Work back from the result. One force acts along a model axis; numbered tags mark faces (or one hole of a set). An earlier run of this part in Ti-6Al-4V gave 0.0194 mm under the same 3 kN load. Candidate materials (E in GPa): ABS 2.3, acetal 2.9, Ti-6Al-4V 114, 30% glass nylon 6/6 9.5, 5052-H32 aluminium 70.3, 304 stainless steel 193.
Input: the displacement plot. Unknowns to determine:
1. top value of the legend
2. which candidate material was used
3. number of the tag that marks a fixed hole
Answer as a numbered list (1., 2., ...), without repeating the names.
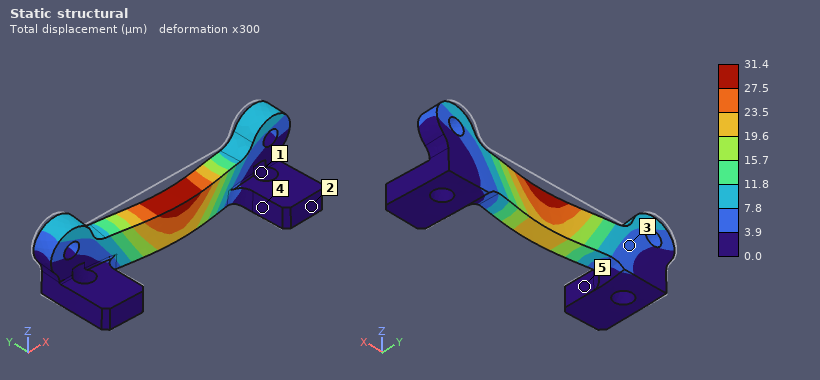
1. 31.4 µm
2. 5052-H32 aluminium
3. 1
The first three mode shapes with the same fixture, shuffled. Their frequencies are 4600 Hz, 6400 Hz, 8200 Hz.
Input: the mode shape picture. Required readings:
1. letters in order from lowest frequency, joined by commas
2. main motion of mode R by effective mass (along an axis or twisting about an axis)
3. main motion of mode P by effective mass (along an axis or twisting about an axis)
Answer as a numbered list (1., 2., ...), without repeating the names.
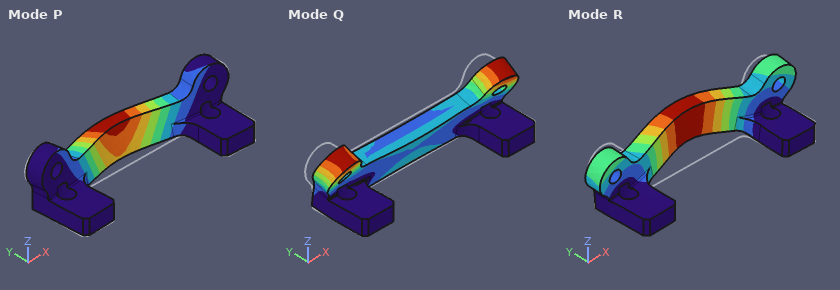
1. P, R, Q
2. along Z
3. along Y
